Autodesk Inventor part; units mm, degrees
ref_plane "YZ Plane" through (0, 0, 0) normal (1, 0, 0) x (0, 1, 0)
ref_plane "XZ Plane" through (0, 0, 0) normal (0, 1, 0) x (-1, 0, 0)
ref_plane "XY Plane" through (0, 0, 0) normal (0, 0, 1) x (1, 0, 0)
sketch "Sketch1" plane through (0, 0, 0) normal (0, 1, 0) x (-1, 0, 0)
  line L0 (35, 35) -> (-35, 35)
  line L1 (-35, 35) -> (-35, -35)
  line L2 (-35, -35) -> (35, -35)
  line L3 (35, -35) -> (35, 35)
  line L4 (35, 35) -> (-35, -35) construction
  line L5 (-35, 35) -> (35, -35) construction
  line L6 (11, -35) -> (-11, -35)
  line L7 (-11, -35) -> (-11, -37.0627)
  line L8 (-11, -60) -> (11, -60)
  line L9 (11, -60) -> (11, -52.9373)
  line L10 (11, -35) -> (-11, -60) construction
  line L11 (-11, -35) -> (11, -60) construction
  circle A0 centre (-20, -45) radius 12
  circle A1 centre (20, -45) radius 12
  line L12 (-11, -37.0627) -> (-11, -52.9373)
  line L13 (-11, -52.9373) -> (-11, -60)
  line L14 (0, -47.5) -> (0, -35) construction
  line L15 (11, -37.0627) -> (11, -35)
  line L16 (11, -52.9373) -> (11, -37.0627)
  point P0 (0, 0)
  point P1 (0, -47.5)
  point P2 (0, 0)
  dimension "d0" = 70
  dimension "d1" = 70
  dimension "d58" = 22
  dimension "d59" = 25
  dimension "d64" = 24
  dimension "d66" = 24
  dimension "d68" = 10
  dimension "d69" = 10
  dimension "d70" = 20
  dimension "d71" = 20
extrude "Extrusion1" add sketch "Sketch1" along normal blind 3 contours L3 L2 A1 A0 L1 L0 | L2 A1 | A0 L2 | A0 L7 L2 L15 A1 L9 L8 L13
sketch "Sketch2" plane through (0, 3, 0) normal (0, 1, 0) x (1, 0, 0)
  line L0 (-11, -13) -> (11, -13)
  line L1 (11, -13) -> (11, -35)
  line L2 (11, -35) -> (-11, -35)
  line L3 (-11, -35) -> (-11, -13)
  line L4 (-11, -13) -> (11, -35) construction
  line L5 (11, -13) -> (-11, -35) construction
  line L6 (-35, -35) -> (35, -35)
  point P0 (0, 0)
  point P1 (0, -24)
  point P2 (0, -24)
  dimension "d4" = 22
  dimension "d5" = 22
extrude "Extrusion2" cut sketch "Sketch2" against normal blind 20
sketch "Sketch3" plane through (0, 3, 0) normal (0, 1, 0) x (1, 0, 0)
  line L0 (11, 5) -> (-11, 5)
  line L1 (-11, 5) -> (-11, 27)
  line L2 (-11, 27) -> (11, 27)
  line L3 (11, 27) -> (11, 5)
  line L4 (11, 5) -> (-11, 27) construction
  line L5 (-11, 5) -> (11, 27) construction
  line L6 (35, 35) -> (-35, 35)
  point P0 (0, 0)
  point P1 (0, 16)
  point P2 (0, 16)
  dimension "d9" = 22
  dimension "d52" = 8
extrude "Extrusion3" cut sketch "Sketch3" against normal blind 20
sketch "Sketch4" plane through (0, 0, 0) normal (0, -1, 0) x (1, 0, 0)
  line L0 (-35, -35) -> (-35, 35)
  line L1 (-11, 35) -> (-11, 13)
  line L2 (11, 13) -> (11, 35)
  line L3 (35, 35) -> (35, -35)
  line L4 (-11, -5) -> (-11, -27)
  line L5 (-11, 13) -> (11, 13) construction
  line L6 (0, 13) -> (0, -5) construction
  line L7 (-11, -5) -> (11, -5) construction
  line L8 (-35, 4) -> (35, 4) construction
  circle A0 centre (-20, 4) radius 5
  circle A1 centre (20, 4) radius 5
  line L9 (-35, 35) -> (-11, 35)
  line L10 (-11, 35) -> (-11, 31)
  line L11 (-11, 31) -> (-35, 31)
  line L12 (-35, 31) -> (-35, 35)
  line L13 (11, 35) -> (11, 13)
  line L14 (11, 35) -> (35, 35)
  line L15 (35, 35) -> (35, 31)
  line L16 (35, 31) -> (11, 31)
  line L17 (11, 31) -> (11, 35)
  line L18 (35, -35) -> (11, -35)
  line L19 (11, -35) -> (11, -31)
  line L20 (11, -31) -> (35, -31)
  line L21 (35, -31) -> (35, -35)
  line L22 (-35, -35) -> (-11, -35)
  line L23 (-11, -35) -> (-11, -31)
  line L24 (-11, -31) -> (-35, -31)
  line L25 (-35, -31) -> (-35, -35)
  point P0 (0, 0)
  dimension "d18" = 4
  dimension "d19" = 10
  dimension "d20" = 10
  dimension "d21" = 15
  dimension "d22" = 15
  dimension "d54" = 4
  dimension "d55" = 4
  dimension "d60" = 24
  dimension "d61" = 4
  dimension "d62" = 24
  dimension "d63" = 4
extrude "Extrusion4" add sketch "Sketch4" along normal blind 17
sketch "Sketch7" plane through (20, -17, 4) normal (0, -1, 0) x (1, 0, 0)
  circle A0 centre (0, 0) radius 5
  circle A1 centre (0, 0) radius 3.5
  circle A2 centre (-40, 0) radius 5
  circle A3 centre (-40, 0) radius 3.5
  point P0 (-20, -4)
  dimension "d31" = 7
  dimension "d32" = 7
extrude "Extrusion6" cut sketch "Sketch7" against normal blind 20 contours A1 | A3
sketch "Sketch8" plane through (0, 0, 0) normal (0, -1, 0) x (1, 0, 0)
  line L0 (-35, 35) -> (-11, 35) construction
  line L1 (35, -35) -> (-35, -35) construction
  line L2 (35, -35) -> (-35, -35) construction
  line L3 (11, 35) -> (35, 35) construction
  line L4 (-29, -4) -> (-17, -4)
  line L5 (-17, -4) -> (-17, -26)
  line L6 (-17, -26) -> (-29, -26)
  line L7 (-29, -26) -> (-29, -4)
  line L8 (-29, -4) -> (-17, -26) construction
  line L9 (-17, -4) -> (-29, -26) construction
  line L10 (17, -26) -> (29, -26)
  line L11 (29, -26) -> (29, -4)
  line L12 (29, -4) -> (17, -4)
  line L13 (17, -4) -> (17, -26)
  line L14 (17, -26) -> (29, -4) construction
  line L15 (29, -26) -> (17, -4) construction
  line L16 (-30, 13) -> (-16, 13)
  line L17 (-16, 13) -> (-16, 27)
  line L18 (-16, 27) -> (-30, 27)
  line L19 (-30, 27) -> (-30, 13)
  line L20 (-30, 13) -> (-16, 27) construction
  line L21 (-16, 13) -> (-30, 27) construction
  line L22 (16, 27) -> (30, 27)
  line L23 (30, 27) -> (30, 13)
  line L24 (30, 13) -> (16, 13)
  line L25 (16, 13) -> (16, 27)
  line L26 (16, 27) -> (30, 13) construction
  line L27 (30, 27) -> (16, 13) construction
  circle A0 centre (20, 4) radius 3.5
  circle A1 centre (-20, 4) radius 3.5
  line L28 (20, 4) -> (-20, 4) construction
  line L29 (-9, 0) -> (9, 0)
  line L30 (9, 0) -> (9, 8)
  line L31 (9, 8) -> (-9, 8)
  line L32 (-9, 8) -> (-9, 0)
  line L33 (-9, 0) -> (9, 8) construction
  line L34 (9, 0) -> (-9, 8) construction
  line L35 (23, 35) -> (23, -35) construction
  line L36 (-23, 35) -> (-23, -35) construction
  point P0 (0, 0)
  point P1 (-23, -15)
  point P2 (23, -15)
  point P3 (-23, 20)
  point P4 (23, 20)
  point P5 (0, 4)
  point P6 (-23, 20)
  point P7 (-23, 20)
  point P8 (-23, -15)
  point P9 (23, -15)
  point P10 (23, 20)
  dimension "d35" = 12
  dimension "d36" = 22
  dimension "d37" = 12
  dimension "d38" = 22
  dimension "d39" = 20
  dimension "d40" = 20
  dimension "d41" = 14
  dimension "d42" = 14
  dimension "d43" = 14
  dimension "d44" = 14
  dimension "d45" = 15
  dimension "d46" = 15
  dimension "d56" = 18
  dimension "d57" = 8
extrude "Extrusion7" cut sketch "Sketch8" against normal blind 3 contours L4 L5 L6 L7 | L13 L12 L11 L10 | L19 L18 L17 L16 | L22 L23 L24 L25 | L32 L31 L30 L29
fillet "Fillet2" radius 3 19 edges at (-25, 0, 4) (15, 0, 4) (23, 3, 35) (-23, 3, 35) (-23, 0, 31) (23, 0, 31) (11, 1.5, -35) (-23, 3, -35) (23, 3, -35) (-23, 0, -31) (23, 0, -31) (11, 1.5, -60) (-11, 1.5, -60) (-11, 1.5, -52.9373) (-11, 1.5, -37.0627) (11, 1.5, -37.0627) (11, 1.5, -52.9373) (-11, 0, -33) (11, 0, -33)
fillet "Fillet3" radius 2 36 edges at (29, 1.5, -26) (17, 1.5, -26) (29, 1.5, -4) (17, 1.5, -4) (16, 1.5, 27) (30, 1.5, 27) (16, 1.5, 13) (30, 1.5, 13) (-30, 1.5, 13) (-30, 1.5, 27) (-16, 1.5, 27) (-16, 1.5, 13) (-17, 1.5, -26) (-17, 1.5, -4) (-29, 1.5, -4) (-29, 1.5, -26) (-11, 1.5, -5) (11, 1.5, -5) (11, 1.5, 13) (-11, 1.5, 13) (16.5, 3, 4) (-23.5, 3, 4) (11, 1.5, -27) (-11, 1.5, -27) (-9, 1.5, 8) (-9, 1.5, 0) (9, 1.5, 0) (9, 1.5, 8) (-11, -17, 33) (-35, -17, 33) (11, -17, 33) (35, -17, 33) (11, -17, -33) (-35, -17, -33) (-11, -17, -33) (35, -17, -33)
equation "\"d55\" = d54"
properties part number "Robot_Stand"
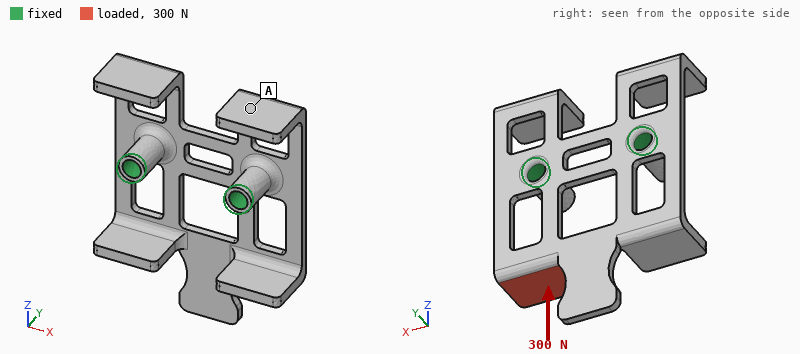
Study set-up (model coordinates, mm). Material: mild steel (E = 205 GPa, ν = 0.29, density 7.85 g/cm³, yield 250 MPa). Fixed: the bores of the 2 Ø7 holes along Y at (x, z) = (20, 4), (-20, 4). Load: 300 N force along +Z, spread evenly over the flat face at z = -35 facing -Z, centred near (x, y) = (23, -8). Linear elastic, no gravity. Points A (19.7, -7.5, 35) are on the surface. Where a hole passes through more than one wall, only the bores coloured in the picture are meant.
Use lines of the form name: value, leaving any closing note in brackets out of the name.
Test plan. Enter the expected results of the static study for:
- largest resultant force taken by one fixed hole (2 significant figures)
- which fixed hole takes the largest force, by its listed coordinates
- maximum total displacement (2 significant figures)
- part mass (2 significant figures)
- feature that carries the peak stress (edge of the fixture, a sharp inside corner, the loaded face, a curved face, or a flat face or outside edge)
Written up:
largest resultant force taken by one fixed hole: 310 N
which fixed hole takes the largest force, by its listed coordinates: (20, 4)
maximum total displacement: 0.36 mm
part mass: 140 g
feature that carries the peak stress: a curved face
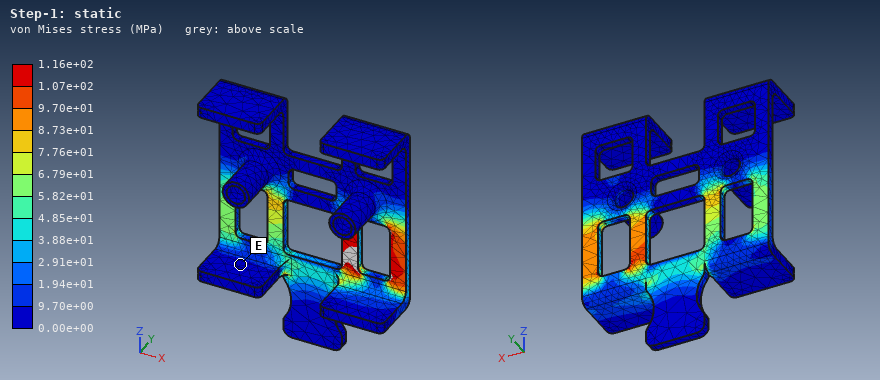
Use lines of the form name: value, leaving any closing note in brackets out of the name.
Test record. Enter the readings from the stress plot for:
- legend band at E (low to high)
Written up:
legend band at E: 0.00e+00 to 9.70e+00 MPa
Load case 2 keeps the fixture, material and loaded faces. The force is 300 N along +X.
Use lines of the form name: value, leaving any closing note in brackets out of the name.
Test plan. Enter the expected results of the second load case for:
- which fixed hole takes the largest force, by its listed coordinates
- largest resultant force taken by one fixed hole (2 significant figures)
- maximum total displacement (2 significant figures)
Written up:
which fixed hole takes the largest force, by its listed coordinates: (20, 4)
largest resultant force taken by one fixed hole: 220 N
maximum total displacement: 0.12 mm
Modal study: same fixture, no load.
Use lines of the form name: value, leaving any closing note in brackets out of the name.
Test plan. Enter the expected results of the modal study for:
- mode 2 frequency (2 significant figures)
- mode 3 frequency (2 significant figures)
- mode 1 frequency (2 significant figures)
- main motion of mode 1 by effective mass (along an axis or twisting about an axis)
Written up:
mode 2 frequency: 1000 Hz
mode 3 frequency: 1000 Hz
mode 1 frequency: 540 Hz
main motion of mode 1 by effective mass: along Y
